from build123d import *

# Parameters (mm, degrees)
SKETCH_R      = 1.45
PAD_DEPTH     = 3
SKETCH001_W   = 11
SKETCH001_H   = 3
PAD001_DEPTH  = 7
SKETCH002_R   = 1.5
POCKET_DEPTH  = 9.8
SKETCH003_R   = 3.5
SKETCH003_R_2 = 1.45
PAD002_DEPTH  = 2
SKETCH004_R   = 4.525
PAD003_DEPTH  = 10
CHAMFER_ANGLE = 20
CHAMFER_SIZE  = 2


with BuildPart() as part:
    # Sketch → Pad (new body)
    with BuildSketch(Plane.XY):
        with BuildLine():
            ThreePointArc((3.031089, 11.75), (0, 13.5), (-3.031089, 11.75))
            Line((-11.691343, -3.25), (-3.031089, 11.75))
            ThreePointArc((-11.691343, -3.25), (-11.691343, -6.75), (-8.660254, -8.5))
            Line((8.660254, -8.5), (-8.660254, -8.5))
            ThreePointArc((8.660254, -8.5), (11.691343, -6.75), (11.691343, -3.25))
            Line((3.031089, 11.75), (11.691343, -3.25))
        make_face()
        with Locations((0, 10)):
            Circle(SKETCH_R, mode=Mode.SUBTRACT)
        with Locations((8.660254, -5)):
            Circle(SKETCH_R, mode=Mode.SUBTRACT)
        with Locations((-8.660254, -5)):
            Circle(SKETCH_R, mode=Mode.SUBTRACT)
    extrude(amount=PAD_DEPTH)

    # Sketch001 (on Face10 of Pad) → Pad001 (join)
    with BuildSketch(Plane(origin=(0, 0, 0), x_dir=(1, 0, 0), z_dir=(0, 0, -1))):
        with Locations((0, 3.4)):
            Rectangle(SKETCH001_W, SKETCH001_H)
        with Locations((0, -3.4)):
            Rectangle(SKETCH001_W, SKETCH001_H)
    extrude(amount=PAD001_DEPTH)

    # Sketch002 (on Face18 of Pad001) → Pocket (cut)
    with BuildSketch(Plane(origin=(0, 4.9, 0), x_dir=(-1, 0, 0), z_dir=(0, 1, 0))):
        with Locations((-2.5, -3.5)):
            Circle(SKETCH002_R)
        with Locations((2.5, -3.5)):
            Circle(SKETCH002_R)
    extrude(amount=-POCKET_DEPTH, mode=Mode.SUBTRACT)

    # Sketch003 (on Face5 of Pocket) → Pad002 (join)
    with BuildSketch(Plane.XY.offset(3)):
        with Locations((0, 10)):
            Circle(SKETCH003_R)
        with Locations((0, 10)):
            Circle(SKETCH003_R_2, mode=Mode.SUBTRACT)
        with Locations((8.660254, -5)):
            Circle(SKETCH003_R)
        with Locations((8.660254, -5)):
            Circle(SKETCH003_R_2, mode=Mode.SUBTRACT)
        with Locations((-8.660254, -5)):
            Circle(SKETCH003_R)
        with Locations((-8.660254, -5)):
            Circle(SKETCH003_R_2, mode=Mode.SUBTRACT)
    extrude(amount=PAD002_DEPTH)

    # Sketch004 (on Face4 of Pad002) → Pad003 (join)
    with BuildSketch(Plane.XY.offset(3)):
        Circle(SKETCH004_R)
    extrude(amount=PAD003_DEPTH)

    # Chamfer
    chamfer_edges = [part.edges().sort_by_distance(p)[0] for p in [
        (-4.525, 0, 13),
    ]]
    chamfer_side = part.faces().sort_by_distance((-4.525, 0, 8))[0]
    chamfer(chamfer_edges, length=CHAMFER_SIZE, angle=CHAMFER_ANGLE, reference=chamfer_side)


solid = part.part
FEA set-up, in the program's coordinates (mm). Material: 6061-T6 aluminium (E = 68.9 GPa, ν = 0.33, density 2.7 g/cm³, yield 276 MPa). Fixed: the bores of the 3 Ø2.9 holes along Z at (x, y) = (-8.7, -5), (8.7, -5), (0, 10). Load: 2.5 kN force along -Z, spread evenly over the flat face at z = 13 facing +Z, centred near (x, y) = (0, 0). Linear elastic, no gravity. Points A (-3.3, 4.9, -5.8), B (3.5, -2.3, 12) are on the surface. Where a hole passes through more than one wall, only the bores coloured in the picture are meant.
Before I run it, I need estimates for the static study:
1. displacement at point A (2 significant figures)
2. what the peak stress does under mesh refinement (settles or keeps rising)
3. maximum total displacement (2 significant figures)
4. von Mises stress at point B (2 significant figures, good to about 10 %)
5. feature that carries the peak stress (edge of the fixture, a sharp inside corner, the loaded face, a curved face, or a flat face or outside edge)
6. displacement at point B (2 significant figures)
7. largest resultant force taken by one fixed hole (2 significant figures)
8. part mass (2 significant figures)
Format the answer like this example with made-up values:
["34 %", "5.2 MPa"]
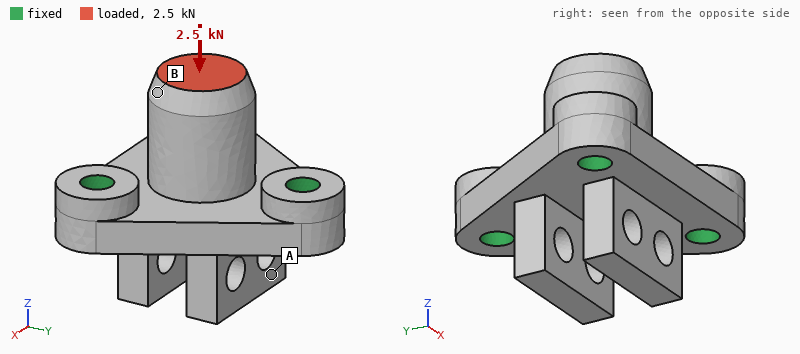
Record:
["12 µm", "keeps rising", "19 µm", "31 MPa", "edge of the fixture", "17 µm", "860 N", "5.9 g"]
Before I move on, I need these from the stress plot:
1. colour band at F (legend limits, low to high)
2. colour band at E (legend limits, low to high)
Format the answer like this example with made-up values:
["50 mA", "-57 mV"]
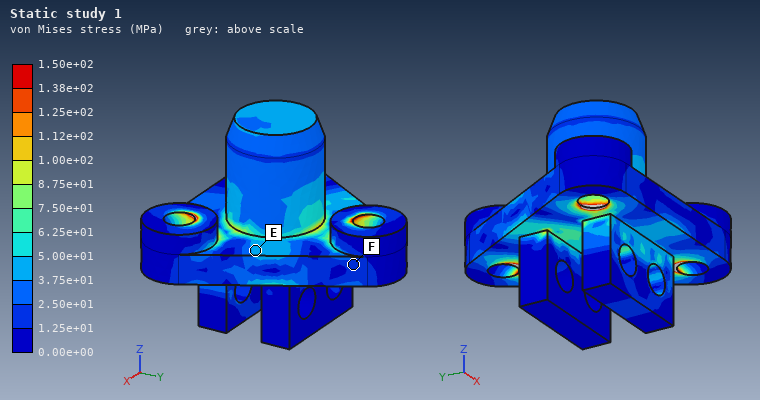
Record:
["1.25e+01 to 2.50e+01 MPa", "3.75e+01 to 5.00e+01 MPa"]
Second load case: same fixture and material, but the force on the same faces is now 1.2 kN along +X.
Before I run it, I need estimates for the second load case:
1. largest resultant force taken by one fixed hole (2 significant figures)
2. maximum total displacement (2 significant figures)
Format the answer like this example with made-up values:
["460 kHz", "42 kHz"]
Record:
["1.0 kN", "66 µm"]
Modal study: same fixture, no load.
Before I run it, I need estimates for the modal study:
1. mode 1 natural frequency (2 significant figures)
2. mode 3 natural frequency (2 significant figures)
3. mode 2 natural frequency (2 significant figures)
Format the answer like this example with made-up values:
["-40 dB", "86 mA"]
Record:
["27 kHz", "31 kHz", "27 kHz"]
